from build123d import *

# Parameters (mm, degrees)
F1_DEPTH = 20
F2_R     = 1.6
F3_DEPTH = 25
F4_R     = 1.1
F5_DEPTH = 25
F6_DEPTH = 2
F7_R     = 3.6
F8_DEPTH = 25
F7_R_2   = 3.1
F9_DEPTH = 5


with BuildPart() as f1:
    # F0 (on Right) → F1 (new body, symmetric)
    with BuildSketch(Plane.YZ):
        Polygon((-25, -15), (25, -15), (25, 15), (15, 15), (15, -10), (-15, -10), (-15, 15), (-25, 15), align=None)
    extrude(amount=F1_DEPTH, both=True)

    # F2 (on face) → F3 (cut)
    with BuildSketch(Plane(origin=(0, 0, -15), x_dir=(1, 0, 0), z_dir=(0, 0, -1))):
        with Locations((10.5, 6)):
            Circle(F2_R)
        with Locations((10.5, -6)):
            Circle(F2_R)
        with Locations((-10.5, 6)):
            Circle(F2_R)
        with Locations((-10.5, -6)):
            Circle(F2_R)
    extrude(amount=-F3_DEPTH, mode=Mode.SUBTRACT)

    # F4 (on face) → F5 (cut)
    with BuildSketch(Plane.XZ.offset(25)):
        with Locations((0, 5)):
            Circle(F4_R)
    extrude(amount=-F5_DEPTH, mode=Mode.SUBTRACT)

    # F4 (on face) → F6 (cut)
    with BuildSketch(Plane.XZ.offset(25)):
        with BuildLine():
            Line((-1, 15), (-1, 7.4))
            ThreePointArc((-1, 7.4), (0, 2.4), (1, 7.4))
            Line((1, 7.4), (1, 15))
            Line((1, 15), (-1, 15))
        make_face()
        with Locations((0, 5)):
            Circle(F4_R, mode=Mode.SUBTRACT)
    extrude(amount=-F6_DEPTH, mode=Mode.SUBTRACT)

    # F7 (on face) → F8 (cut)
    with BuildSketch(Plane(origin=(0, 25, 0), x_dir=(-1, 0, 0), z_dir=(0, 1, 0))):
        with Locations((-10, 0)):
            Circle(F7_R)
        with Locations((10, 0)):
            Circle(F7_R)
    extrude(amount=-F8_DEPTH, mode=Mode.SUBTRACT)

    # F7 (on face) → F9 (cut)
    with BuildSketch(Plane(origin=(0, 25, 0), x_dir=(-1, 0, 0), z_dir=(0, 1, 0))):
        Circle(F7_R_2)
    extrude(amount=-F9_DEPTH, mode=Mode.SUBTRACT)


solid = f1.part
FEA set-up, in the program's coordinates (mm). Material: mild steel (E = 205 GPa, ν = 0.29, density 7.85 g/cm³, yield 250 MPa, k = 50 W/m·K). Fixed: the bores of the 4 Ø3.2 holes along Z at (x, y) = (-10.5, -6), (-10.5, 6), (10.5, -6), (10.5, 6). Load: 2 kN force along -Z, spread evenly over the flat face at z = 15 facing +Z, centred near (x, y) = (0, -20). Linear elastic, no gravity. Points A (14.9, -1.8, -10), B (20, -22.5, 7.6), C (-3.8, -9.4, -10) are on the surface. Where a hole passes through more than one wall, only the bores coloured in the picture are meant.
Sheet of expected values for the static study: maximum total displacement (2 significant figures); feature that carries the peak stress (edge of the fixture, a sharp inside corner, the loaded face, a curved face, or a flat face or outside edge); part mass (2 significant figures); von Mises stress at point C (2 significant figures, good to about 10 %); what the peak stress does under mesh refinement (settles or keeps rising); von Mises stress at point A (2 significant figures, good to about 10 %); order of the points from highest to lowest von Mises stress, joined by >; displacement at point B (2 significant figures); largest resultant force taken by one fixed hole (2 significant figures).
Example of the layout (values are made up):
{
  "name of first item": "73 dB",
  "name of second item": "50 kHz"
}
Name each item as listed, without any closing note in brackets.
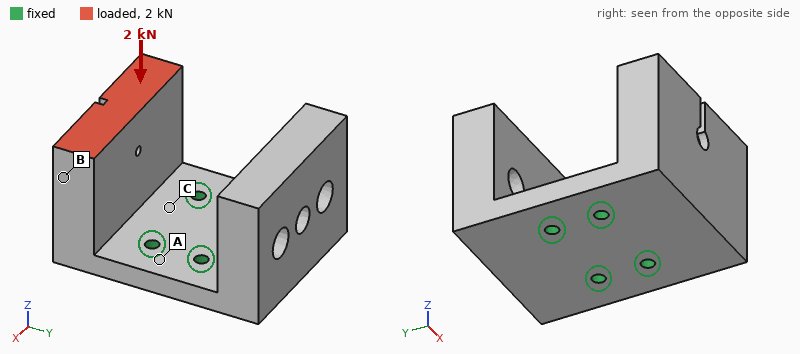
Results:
{
  "maximum total displacement": "76 µm",
  "feature that carries the peak stress": "edge of the fixture",
  "part mass": "230 g",
  "von Mises stress at point C": "91 MPa",
  "what the peak stress does under mesh refinement": "keeps rising",
  "von Mises stress at point A": "34 MPa",
  "order of the points from highest to lowest von Mises stress, joined by >": "C > A > B",
  "displacement at point B": "58 µm",
  "largest resultant force taken by one fixed hole": "1.4 kN"
}
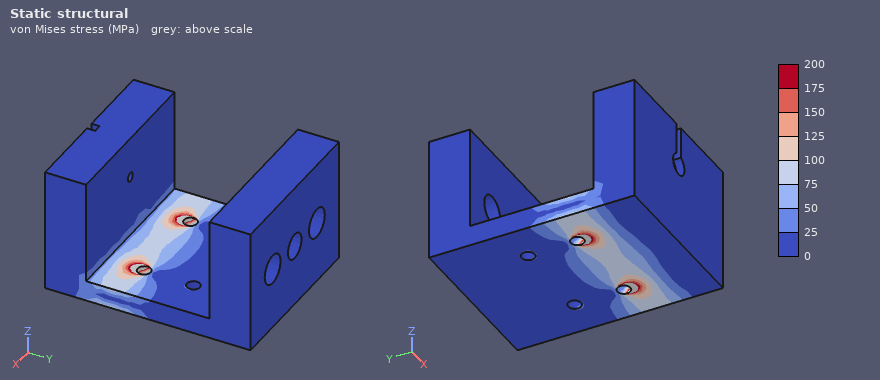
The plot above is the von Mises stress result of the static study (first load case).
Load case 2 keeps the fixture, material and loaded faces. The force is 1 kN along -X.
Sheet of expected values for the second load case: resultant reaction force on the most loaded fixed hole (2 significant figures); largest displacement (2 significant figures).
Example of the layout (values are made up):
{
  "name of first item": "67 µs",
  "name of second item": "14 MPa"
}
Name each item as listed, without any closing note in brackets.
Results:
{
  "resultant reaction force on the most loaded fixed hole": "1.3 kN",
  "largest displacement": "24 µm"
}
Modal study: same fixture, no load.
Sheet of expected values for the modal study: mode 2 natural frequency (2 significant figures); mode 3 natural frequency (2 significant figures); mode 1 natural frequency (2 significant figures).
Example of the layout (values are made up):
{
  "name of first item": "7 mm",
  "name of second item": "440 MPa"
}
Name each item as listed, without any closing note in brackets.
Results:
{
  "mode 2 natural frequency": "2500 Hz",
  "mode 3 natural frequency": "5400 Hz",
  "mode 1 natural frequency": "2400 Hz"
}
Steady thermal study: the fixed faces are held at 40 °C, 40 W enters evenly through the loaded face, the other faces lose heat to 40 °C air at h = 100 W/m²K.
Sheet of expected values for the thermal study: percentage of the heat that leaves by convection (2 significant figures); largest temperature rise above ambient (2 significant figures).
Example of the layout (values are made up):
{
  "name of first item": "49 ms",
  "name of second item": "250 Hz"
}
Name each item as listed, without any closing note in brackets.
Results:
{
  "percentage of the heat that leaves by convection": "44 %",
  "largest temperature rise above ambient": "74 K"
}
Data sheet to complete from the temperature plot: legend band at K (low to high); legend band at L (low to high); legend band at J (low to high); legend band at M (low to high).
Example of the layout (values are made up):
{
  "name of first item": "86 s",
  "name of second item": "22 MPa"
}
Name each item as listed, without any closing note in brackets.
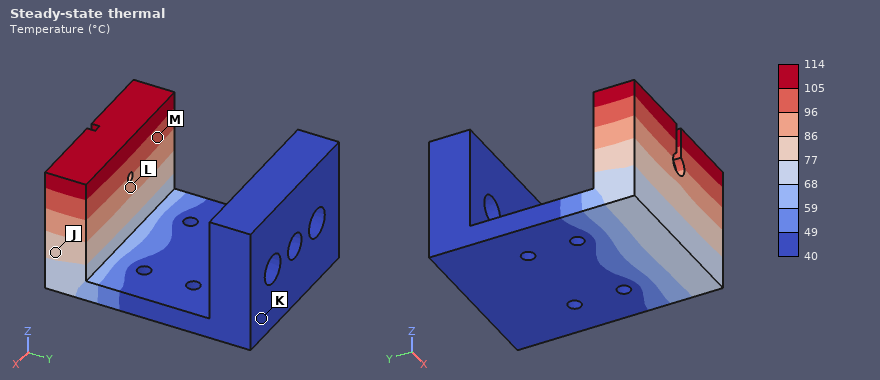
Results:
{
  "legend band at K": "40 to 49 °C",
  "legend band at L": "86 to 96 °C",
  "legend band at J": "77 to 86 °C",
  "legend band at M": "96 to 105 °C"
}
